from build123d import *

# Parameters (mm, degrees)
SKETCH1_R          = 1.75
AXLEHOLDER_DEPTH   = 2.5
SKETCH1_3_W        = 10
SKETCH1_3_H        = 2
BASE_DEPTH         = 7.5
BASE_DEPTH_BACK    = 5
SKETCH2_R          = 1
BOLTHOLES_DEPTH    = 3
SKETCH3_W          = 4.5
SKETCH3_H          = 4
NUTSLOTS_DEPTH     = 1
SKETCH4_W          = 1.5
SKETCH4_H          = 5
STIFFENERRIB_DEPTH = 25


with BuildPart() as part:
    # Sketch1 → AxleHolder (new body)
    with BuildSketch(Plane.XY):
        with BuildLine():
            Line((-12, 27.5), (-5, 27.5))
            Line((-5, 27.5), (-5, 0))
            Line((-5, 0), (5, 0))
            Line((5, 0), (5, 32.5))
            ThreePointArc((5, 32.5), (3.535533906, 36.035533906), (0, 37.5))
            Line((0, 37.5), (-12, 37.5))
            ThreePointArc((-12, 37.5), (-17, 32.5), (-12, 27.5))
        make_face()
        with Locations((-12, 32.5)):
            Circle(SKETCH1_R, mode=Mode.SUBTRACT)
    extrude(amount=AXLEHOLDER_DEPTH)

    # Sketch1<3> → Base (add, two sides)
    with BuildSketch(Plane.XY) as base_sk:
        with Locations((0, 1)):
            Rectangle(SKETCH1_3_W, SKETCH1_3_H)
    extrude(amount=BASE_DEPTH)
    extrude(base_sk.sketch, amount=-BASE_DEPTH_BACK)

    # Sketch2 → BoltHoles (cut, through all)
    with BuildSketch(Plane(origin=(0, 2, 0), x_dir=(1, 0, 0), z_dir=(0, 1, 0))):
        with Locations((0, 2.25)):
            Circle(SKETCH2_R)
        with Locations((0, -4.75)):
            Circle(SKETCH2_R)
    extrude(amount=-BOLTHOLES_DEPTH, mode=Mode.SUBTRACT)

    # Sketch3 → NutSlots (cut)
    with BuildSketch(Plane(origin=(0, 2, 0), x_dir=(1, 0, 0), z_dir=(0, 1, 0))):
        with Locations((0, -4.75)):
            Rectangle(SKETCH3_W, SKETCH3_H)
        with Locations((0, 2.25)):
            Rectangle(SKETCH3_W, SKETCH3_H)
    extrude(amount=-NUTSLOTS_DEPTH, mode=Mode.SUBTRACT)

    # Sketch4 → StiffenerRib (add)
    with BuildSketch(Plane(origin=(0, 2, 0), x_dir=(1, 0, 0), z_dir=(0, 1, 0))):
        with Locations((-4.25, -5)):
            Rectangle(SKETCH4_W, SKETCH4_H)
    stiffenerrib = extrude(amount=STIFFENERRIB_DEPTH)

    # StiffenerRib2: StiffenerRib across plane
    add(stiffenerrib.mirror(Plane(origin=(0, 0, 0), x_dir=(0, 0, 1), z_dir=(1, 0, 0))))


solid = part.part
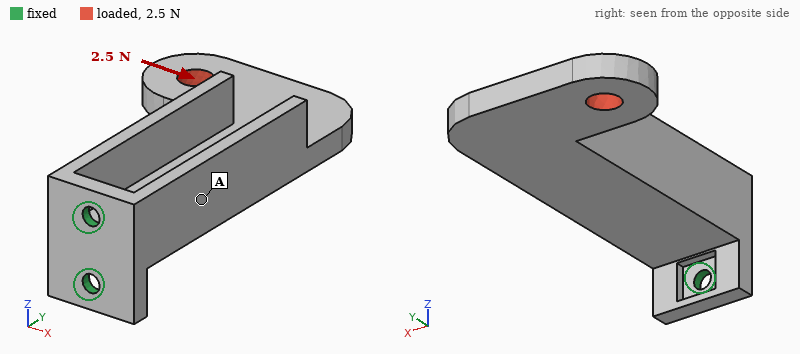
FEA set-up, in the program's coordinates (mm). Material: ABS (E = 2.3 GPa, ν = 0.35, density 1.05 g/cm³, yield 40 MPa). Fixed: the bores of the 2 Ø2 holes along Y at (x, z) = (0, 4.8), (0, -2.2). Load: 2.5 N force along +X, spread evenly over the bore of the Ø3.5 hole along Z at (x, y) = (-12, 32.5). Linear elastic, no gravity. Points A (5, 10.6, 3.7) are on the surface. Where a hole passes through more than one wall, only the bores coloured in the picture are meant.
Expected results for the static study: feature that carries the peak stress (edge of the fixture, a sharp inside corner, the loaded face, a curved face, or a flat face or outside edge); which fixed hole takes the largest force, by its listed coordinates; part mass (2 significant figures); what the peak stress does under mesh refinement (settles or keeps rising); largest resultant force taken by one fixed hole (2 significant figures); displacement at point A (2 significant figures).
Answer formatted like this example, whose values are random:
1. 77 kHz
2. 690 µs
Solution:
1. edge of the fixture
2. (0, -2.2)
3. 1.8 g
4. keeps rising
5. 1.6 N
6. 0.13 mm
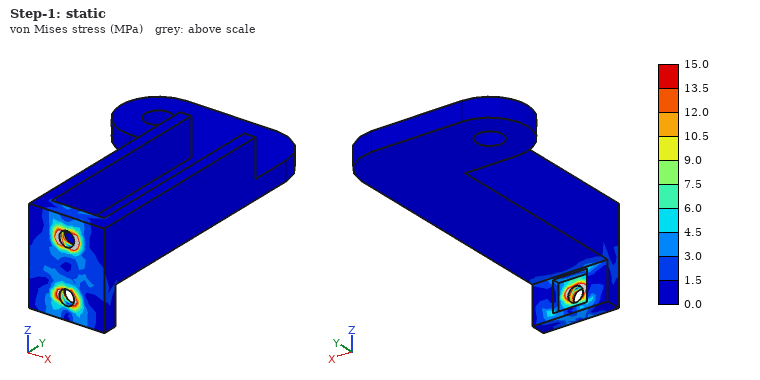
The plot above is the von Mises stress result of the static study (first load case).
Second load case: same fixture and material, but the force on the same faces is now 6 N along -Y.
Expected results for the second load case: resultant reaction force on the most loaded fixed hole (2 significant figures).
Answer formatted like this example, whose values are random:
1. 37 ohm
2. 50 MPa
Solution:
1. 3.3 N
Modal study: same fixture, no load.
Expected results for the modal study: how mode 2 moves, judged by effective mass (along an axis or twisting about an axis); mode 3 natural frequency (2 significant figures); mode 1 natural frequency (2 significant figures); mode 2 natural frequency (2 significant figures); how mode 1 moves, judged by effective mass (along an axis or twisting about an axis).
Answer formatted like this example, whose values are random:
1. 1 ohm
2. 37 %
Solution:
1. along Z
2. 1400 Hz
3. 450 Hz
4. 630 Hz
5. along X
